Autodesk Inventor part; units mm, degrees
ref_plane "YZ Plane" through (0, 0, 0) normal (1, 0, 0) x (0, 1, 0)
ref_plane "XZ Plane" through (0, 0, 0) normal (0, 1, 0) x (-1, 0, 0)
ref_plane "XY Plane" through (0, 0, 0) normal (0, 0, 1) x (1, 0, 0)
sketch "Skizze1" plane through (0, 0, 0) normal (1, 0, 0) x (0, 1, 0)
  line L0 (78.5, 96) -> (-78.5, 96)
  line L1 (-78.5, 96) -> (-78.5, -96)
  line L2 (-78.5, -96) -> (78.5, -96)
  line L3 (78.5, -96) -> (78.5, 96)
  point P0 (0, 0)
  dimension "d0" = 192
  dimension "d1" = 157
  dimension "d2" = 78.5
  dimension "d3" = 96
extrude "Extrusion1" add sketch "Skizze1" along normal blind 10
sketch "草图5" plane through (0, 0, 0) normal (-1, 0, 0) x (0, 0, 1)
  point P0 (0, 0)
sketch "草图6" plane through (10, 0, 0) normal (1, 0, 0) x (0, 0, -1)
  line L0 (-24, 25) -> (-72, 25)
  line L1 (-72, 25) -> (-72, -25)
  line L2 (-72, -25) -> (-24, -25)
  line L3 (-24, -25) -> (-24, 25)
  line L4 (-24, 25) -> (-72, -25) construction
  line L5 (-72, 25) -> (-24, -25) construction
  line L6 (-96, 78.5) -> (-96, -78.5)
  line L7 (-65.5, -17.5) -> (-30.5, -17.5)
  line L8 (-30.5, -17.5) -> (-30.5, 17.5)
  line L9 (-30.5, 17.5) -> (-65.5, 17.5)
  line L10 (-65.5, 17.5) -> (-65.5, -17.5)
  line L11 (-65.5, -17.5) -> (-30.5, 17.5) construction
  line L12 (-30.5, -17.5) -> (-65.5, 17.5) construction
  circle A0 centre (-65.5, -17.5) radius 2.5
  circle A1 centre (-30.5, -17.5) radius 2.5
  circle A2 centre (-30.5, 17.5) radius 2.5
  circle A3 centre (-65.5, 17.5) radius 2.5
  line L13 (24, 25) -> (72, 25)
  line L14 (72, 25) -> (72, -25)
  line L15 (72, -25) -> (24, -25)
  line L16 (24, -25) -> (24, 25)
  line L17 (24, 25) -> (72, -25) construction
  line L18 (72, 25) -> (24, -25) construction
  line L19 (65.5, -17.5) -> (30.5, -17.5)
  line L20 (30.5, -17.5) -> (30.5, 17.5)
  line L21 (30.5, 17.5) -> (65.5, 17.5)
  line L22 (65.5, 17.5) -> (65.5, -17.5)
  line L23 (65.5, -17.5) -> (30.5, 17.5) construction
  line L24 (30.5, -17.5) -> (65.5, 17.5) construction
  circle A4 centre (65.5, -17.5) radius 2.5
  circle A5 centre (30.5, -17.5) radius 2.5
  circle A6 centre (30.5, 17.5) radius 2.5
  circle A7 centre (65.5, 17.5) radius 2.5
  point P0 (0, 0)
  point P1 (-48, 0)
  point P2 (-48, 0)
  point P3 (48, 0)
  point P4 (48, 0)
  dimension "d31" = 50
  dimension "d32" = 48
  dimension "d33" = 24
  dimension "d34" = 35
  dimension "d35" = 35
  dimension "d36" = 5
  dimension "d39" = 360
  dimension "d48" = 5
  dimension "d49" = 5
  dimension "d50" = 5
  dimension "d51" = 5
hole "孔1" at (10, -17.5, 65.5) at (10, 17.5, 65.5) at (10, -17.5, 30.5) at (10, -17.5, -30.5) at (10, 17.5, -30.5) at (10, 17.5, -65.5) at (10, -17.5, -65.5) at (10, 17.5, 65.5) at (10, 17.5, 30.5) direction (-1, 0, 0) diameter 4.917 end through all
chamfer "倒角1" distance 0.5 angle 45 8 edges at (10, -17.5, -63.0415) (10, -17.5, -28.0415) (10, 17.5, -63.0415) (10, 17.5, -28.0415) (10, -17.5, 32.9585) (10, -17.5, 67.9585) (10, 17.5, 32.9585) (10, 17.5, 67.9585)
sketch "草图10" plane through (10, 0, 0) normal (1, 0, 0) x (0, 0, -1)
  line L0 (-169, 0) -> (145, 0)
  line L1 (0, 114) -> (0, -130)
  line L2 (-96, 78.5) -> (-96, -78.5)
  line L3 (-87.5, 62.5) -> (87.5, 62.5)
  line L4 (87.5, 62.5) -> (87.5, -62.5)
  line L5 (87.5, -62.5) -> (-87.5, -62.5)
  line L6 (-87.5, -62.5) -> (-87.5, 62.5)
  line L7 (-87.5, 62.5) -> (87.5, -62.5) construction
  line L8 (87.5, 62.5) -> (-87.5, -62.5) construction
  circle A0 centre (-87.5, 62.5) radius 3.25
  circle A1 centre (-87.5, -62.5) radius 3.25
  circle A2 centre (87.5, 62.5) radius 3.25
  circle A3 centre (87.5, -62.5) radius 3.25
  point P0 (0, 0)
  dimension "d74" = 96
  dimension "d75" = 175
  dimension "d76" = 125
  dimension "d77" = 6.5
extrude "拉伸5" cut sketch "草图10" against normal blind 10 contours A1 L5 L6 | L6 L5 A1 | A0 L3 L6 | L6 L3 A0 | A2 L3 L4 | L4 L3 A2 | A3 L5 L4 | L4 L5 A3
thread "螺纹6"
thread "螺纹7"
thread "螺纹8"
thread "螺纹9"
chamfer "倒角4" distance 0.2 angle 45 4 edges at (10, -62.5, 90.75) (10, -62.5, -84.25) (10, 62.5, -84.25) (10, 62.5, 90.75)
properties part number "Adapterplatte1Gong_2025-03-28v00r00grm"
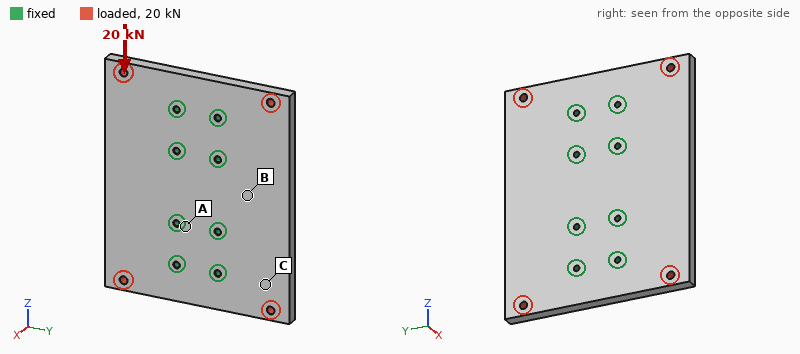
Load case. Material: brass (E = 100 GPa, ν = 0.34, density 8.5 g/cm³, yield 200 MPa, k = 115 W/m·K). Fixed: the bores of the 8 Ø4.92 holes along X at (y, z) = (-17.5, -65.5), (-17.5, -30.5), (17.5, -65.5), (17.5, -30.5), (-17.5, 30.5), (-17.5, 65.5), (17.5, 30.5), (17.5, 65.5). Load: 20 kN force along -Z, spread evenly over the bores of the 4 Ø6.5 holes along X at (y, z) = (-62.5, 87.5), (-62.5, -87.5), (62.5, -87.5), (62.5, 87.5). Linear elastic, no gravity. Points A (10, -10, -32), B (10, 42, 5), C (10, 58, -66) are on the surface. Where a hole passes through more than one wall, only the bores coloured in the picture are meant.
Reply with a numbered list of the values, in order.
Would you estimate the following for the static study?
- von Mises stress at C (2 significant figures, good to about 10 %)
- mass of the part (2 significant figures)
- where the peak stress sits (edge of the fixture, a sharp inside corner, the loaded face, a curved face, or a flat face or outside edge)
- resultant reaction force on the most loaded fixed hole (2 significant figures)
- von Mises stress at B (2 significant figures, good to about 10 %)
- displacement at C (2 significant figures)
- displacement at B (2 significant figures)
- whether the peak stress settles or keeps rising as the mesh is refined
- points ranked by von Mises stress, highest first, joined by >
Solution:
1. 14 MPa
2. 2.5 kg
3. edge of the fixture
4. 2.8 kN
5. 9.5 MPa
6. 9.5 µm
7. 4.4 µm
8. keeps rising
9. C > B > A
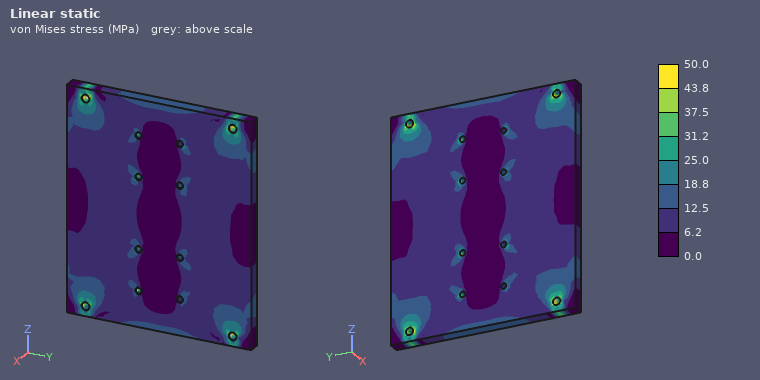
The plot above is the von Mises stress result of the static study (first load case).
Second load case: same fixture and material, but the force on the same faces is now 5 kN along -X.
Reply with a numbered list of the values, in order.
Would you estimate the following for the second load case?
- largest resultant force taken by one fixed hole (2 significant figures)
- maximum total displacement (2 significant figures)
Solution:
1. 1.5 kN
2. 0.17 mm
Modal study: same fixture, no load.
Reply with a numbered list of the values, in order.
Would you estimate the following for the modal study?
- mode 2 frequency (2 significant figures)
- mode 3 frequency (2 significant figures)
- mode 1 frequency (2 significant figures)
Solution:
1. 1400 Hz
2. 1600 Hz
3. 1300 Hz
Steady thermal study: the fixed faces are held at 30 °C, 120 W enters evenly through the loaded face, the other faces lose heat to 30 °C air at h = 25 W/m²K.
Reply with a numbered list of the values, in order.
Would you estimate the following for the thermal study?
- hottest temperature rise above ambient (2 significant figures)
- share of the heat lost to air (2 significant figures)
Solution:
1. 31 K
2. 12 %
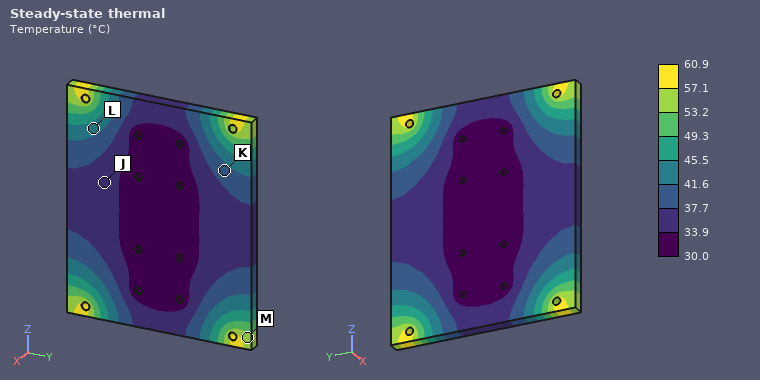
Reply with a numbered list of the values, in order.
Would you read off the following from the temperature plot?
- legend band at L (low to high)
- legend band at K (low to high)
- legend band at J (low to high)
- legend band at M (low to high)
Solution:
1. 41.6 to 45.5 °C
2. 37.7 to 41.6 °C
3. 33.9 to 37.7 °C
4. 53.2 to 57.1 °C
